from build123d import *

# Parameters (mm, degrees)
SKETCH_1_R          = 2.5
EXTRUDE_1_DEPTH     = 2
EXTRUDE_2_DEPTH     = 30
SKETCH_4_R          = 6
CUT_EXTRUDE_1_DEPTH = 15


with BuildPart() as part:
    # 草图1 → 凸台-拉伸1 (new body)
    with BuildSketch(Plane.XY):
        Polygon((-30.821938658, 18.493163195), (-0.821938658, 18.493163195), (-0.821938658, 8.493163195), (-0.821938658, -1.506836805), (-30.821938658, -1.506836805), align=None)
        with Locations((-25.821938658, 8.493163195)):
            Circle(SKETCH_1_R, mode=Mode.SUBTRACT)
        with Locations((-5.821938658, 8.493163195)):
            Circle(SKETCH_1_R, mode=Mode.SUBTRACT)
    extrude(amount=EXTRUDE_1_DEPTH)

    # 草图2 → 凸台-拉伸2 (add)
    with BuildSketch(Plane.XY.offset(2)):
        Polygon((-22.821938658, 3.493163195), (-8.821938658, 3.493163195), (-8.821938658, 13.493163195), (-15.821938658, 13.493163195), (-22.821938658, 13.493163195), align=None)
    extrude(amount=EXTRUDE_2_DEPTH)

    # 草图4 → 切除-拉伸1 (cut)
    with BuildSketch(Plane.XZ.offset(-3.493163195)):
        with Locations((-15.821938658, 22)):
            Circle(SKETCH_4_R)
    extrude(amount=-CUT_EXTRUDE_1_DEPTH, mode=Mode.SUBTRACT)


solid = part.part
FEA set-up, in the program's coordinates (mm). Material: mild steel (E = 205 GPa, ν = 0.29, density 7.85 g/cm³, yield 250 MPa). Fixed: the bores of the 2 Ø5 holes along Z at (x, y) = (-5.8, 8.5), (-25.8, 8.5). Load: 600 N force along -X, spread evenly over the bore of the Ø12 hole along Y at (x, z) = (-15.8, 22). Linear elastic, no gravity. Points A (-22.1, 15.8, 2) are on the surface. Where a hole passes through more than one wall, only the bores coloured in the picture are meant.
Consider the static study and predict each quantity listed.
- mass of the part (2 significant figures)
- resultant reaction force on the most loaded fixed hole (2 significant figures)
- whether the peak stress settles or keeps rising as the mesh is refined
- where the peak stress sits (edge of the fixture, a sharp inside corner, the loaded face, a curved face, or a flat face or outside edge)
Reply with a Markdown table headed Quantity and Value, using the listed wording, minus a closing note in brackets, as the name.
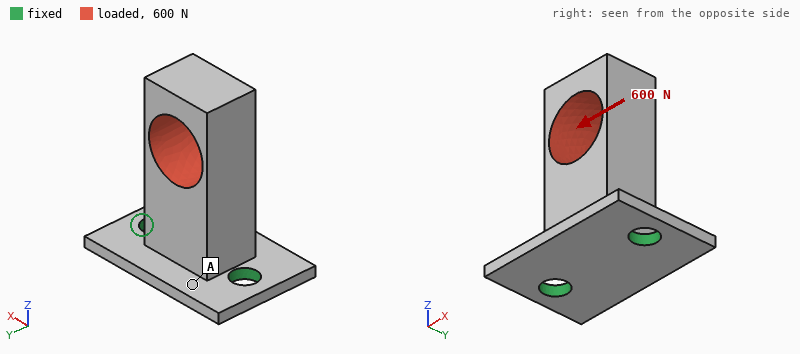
| Quantity | Value |
|---|---|
| mass of the part | 33 g |
| resultant reaction force on the most loaded fixed hole | 900 N |
| whether the peak stress settles or keeps rising as the mesh is refined | keeps rising |
| where the peak stress sits | a sharp inside corner |
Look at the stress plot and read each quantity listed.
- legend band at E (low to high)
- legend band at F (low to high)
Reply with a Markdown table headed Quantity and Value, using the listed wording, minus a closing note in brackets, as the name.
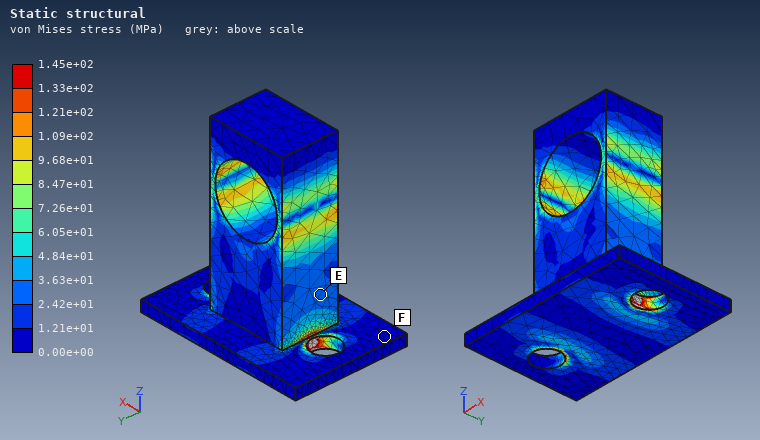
| Quantity | Value |
|---|---|
| legend band at E | 2.42e+01 to 3.63e+01 MPa |
| legend band at F | 0.00e+00 to 1.21e+01 MPa |
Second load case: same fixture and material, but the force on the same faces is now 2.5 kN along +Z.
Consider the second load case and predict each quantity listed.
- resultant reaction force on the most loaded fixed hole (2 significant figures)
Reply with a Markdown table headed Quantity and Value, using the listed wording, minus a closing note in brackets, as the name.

| Quantity | Value |
|---|---|
| resultant reaction force on the most loaded fixed hole | 1.4 kN |
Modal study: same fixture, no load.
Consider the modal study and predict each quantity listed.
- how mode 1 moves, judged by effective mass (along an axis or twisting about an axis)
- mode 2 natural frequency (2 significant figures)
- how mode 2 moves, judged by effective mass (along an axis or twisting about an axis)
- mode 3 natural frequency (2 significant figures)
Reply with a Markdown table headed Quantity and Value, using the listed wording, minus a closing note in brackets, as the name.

| Quantity | Value |
|---|---|
| how mode 1 moves, judged by effective mass | along Y |
| mode 2 natural frequency | 6700 Hz |
| how mode 2 moves, judged by effective mass | along X |
| mode 3 natural frequency | 18 kHz |
